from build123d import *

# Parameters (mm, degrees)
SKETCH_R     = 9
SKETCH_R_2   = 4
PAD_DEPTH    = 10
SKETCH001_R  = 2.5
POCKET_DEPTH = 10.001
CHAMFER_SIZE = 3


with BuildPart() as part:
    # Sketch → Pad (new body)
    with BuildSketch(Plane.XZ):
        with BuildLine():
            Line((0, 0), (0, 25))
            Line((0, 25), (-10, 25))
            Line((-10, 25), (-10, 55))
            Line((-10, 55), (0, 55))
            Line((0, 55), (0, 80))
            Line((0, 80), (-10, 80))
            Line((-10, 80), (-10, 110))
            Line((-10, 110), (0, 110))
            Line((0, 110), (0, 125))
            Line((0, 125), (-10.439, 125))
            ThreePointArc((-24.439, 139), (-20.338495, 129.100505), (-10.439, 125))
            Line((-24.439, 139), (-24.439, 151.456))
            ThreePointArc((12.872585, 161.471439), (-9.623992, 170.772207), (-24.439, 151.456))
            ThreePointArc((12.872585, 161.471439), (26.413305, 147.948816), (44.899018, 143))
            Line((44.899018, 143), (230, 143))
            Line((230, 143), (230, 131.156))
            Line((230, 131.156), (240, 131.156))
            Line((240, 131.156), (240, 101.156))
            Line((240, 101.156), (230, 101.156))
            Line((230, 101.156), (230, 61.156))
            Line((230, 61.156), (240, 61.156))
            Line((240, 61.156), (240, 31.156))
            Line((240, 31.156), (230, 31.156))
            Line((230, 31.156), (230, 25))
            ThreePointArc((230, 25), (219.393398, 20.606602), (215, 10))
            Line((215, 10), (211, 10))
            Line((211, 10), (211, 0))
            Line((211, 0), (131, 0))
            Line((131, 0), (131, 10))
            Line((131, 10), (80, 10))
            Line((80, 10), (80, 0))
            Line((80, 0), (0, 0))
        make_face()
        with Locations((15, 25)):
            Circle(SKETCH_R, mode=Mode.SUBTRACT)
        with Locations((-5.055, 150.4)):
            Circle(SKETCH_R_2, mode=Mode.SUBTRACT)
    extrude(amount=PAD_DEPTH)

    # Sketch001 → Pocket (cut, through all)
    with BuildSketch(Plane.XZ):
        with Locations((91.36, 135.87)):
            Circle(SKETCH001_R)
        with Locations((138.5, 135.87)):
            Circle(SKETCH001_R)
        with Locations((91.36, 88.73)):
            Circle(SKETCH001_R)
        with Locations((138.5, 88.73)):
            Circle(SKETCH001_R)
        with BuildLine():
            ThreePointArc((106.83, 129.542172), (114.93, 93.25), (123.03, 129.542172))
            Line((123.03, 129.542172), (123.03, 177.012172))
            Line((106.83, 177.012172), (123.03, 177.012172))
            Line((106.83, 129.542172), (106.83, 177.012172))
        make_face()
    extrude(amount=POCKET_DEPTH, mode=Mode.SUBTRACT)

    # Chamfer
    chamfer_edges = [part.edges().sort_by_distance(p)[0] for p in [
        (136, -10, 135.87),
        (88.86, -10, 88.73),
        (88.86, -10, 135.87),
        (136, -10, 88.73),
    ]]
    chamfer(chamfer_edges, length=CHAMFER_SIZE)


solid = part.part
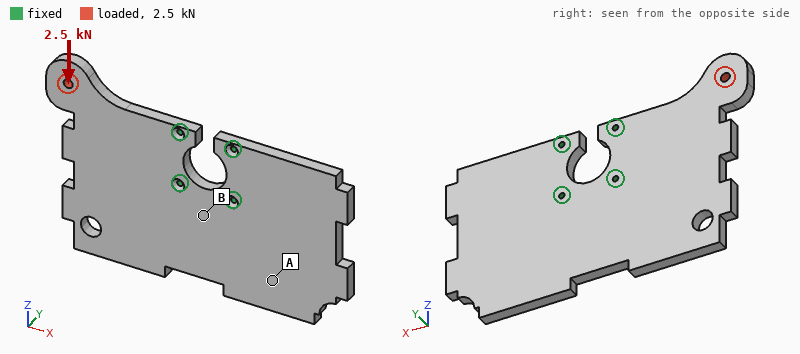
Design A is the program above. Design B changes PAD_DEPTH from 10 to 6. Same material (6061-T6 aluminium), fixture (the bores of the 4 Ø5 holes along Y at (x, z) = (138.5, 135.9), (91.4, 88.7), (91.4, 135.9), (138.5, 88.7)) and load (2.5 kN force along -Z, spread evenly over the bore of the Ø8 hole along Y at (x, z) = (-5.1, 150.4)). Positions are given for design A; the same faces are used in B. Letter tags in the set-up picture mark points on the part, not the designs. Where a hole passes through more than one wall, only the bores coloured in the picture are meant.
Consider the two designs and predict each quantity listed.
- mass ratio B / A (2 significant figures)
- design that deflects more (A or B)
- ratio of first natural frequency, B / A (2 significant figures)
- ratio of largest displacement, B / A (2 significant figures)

0.60
B
0.61
1.8
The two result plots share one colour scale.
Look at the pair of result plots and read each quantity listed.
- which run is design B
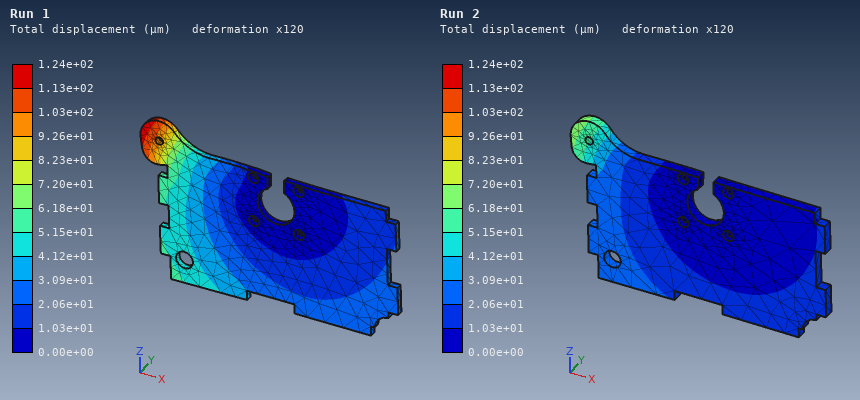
Run 1
